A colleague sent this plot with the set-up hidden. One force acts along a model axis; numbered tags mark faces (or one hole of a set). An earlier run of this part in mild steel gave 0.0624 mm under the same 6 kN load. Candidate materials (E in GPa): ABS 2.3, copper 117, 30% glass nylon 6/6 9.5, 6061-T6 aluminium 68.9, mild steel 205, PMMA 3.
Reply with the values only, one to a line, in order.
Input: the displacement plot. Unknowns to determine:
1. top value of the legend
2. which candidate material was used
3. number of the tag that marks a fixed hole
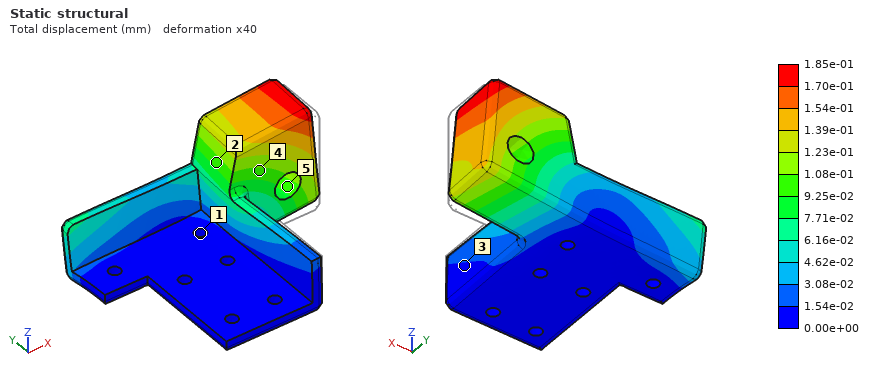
1.85e-01 mm
6061-T6 aluminium
1
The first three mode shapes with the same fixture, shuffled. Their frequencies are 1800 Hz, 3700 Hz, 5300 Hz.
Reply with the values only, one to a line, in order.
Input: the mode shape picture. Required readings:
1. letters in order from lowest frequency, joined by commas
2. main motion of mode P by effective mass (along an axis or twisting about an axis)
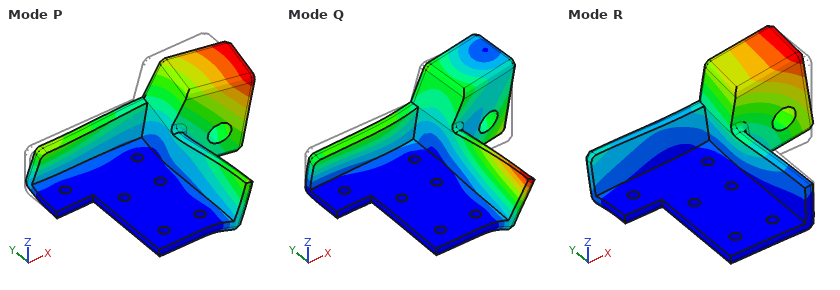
R, P, Q
along Y
